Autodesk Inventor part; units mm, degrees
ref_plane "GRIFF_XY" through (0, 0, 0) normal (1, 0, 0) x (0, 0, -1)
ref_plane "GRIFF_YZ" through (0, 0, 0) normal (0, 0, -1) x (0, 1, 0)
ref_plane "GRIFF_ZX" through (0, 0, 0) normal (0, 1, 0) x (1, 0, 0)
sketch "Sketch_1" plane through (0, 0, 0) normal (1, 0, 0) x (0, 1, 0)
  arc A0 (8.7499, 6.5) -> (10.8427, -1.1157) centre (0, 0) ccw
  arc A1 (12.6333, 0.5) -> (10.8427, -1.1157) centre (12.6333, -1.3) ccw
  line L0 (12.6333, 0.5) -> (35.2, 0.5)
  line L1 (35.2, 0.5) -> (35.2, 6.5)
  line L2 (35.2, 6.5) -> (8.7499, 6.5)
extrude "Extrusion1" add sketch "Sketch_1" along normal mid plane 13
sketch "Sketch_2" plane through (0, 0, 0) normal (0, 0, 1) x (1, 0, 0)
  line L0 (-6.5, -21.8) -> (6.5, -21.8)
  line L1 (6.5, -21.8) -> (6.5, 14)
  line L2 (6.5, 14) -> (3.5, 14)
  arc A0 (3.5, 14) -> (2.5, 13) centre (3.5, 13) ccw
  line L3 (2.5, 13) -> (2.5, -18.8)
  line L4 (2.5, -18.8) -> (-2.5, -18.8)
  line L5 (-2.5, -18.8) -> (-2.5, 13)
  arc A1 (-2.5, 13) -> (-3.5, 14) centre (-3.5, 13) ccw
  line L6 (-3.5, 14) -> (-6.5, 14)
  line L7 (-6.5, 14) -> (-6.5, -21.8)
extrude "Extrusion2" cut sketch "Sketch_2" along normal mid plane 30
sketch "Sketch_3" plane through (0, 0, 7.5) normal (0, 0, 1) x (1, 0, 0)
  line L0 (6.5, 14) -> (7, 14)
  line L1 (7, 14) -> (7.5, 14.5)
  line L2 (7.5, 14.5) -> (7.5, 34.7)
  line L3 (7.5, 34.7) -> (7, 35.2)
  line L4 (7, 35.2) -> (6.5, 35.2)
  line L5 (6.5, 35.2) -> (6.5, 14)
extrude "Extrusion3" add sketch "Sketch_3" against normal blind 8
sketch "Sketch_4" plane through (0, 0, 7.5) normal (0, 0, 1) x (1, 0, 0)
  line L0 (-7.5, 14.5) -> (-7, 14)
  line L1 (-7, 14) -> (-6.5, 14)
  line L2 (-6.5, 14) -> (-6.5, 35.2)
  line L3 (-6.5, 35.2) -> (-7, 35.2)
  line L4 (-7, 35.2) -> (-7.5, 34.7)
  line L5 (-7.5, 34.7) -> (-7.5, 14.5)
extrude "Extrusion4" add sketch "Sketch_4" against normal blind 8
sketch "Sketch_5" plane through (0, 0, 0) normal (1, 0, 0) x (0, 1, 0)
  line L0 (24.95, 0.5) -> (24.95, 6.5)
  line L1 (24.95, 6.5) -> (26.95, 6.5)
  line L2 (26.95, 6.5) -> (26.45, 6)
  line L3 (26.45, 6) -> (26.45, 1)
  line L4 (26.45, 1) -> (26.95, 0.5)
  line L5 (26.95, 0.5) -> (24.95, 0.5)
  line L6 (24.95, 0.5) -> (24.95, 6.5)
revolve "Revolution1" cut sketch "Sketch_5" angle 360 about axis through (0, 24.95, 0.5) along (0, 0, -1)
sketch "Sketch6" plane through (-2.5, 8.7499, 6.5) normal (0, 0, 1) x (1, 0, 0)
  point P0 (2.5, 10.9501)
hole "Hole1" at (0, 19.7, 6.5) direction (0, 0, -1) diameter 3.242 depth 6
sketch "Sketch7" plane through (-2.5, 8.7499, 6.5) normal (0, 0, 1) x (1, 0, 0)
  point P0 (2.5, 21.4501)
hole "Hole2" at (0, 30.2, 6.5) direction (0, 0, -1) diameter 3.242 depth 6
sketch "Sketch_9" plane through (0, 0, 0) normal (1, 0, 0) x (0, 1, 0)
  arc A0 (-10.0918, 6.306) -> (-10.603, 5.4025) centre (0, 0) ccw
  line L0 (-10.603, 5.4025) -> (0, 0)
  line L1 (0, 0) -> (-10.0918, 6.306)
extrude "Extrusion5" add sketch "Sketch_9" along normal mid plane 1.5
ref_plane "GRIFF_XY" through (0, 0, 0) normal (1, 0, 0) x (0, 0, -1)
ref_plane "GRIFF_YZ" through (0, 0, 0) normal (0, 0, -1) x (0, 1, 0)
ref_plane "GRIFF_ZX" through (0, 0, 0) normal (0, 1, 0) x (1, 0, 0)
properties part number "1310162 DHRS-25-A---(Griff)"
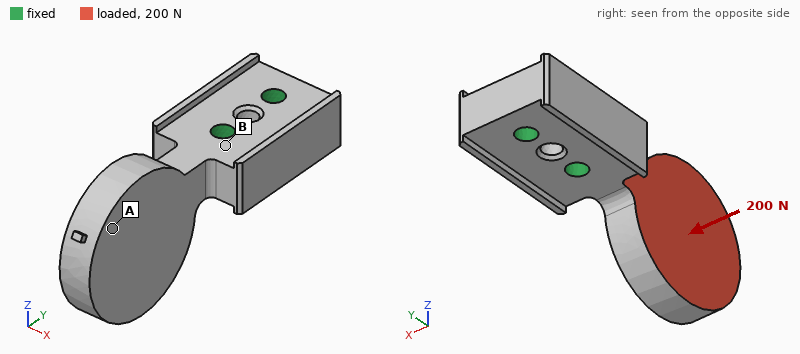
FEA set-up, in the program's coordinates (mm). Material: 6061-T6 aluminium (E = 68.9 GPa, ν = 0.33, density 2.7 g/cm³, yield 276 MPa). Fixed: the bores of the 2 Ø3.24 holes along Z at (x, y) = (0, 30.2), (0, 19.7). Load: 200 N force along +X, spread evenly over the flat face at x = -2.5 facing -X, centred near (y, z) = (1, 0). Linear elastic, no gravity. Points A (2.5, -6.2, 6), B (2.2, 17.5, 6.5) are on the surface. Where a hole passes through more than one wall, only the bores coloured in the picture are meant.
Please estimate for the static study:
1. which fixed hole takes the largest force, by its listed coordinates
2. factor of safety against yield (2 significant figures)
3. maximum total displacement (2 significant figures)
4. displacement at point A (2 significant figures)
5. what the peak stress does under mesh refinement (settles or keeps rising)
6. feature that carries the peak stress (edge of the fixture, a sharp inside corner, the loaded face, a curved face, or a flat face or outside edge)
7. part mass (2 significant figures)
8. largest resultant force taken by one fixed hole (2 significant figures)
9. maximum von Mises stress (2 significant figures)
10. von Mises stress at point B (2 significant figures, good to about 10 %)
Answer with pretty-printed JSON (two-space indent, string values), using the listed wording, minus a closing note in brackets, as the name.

{
  "which fixed hole takes the largest force, by its listed coordinates": "(0, 19.7)",
  "factor of safety against yield": "1.5",
  "maximum total displacement": "0.11 mm",
  "displacement at point A": "0.078 mm",
  "what the peak stress does under mesh refinement": "settles",
  "feature that carries the peak stress": "a curved face",
  "part mass": "10 g",
  "largest resultant force taken by one fixed hole": "400 N",
  "maximum von Mises stress": "180 MPa",
  "von Mises stress at point B": "27 MPa"
}
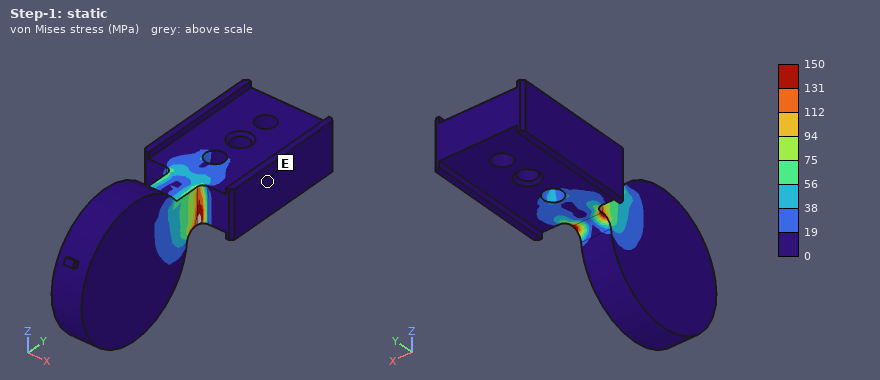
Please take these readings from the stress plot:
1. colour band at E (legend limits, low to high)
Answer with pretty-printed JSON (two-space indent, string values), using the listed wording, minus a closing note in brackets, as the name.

{
  "colour band at E": "0 to 19 MPa"
}
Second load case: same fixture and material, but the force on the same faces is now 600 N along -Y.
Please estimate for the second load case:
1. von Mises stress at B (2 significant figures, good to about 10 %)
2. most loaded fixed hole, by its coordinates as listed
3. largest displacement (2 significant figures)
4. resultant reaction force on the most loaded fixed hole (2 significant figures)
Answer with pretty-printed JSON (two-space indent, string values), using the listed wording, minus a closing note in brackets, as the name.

{
  "von Mises stress at B": "29 MPa",
  "most loaded fixed hole, by its coordinates as listed": "(0, 19.7)",
  "largest displacement": "97 µm",
  "resultant reaction force on the most loaded fixed hole": "540 N"
}
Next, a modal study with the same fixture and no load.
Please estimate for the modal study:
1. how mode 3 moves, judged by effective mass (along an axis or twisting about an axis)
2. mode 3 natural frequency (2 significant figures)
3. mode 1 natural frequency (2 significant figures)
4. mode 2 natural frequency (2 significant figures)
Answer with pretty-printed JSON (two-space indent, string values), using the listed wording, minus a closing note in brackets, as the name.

{
  "how mode 3 moves, judged by effective mass": "twisting about Y",
  "mode 3 natural frequency": "8300 Hz",
  "mode 1 natural frequency": "3700 Hz",
  "mode 2 natural frequency": "3800 Hz"
}
